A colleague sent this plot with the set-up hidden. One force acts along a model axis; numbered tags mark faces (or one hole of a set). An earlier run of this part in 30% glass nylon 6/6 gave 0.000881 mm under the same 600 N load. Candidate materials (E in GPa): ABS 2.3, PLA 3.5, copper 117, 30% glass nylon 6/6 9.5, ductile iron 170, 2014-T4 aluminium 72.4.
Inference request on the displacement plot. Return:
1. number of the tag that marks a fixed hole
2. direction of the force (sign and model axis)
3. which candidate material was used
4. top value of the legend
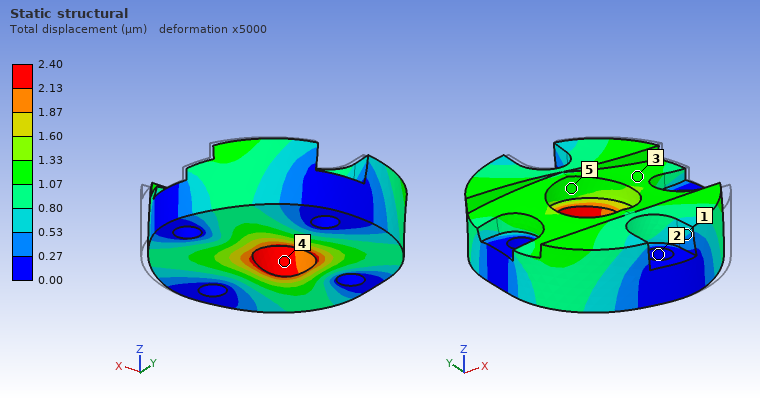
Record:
2
-X
PLA
2.40 µm
